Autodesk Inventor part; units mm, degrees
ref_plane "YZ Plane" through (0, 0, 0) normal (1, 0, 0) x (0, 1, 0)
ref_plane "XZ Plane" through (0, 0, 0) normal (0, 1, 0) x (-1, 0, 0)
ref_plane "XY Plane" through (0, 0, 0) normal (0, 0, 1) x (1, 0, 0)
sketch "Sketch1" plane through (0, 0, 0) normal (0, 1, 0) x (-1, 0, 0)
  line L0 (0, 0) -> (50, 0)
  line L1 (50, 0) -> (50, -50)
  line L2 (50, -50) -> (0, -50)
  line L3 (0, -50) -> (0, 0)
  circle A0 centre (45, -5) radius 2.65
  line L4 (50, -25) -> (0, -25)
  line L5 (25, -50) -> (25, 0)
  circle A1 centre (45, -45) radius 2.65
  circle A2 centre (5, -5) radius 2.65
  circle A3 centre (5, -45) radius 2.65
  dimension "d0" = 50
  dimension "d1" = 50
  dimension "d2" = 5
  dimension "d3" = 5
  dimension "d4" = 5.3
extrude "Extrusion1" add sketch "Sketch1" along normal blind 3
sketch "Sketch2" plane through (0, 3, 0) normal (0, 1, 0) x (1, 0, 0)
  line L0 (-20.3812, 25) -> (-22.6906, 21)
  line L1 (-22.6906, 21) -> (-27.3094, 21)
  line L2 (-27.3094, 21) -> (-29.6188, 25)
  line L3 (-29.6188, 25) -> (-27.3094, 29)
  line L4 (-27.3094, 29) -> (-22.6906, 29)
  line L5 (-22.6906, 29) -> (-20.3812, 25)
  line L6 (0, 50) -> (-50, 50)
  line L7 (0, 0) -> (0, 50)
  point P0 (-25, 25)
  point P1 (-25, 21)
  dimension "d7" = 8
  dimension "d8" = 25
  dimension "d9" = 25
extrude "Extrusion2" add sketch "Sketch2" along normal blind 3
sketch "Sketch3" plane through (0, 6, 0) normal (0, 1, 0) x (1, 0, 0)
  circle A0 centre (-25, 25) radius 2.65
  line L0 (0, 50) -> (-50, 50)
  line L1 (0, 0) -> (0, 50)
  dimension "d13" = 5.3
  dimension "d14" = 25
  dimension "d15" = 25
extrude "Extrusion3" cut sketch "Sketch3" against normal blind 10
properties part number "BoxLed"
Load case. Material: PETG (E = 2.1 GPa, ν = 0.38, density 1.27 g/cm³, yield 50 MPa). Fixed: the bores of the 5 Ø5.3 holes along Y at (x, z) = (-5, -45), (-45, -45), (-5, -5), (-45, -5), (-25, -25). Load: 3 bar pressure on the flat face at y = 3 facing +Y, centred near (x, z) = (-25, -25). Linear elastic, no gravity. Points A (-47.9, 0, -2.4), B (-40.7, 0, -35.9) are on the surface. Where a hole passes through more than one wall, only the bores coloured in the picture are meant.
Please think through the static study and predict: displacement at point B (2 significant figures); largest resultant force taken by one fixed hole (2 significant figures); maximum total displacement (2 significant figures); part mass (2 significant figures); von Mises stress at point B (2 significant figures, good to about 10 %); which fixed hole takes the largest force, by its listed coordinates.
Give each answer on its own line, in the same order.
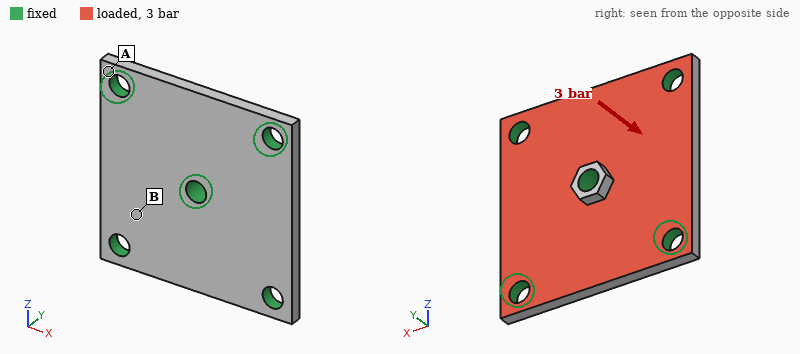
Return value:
0.091 mm
240 N
0.25 mm
9.2 g
6.5 MPa
(-25, -25)
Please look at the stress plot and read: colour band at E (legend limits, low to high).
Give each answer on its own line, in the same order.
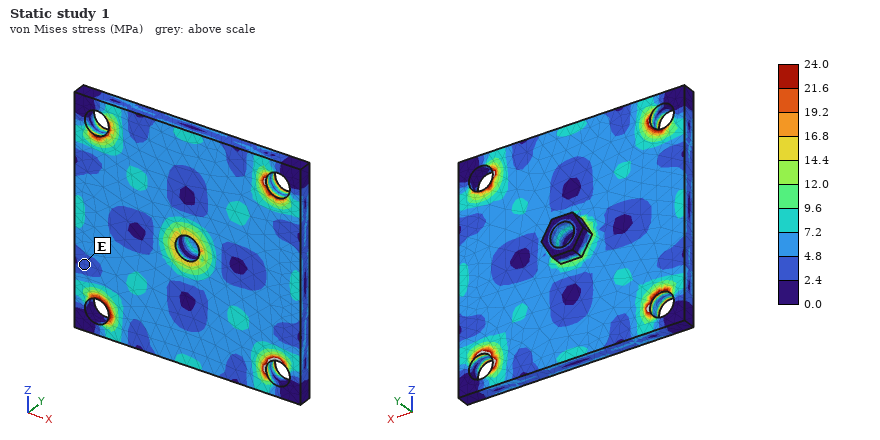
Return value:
2.4 to 4.8 MPa
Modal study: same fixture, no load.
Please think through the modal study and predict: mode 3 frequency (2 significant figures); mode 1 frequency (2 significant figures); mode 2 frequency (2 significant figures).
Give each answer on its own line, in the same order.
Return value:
3500 Hz
3300 Hz
3500 Hz
